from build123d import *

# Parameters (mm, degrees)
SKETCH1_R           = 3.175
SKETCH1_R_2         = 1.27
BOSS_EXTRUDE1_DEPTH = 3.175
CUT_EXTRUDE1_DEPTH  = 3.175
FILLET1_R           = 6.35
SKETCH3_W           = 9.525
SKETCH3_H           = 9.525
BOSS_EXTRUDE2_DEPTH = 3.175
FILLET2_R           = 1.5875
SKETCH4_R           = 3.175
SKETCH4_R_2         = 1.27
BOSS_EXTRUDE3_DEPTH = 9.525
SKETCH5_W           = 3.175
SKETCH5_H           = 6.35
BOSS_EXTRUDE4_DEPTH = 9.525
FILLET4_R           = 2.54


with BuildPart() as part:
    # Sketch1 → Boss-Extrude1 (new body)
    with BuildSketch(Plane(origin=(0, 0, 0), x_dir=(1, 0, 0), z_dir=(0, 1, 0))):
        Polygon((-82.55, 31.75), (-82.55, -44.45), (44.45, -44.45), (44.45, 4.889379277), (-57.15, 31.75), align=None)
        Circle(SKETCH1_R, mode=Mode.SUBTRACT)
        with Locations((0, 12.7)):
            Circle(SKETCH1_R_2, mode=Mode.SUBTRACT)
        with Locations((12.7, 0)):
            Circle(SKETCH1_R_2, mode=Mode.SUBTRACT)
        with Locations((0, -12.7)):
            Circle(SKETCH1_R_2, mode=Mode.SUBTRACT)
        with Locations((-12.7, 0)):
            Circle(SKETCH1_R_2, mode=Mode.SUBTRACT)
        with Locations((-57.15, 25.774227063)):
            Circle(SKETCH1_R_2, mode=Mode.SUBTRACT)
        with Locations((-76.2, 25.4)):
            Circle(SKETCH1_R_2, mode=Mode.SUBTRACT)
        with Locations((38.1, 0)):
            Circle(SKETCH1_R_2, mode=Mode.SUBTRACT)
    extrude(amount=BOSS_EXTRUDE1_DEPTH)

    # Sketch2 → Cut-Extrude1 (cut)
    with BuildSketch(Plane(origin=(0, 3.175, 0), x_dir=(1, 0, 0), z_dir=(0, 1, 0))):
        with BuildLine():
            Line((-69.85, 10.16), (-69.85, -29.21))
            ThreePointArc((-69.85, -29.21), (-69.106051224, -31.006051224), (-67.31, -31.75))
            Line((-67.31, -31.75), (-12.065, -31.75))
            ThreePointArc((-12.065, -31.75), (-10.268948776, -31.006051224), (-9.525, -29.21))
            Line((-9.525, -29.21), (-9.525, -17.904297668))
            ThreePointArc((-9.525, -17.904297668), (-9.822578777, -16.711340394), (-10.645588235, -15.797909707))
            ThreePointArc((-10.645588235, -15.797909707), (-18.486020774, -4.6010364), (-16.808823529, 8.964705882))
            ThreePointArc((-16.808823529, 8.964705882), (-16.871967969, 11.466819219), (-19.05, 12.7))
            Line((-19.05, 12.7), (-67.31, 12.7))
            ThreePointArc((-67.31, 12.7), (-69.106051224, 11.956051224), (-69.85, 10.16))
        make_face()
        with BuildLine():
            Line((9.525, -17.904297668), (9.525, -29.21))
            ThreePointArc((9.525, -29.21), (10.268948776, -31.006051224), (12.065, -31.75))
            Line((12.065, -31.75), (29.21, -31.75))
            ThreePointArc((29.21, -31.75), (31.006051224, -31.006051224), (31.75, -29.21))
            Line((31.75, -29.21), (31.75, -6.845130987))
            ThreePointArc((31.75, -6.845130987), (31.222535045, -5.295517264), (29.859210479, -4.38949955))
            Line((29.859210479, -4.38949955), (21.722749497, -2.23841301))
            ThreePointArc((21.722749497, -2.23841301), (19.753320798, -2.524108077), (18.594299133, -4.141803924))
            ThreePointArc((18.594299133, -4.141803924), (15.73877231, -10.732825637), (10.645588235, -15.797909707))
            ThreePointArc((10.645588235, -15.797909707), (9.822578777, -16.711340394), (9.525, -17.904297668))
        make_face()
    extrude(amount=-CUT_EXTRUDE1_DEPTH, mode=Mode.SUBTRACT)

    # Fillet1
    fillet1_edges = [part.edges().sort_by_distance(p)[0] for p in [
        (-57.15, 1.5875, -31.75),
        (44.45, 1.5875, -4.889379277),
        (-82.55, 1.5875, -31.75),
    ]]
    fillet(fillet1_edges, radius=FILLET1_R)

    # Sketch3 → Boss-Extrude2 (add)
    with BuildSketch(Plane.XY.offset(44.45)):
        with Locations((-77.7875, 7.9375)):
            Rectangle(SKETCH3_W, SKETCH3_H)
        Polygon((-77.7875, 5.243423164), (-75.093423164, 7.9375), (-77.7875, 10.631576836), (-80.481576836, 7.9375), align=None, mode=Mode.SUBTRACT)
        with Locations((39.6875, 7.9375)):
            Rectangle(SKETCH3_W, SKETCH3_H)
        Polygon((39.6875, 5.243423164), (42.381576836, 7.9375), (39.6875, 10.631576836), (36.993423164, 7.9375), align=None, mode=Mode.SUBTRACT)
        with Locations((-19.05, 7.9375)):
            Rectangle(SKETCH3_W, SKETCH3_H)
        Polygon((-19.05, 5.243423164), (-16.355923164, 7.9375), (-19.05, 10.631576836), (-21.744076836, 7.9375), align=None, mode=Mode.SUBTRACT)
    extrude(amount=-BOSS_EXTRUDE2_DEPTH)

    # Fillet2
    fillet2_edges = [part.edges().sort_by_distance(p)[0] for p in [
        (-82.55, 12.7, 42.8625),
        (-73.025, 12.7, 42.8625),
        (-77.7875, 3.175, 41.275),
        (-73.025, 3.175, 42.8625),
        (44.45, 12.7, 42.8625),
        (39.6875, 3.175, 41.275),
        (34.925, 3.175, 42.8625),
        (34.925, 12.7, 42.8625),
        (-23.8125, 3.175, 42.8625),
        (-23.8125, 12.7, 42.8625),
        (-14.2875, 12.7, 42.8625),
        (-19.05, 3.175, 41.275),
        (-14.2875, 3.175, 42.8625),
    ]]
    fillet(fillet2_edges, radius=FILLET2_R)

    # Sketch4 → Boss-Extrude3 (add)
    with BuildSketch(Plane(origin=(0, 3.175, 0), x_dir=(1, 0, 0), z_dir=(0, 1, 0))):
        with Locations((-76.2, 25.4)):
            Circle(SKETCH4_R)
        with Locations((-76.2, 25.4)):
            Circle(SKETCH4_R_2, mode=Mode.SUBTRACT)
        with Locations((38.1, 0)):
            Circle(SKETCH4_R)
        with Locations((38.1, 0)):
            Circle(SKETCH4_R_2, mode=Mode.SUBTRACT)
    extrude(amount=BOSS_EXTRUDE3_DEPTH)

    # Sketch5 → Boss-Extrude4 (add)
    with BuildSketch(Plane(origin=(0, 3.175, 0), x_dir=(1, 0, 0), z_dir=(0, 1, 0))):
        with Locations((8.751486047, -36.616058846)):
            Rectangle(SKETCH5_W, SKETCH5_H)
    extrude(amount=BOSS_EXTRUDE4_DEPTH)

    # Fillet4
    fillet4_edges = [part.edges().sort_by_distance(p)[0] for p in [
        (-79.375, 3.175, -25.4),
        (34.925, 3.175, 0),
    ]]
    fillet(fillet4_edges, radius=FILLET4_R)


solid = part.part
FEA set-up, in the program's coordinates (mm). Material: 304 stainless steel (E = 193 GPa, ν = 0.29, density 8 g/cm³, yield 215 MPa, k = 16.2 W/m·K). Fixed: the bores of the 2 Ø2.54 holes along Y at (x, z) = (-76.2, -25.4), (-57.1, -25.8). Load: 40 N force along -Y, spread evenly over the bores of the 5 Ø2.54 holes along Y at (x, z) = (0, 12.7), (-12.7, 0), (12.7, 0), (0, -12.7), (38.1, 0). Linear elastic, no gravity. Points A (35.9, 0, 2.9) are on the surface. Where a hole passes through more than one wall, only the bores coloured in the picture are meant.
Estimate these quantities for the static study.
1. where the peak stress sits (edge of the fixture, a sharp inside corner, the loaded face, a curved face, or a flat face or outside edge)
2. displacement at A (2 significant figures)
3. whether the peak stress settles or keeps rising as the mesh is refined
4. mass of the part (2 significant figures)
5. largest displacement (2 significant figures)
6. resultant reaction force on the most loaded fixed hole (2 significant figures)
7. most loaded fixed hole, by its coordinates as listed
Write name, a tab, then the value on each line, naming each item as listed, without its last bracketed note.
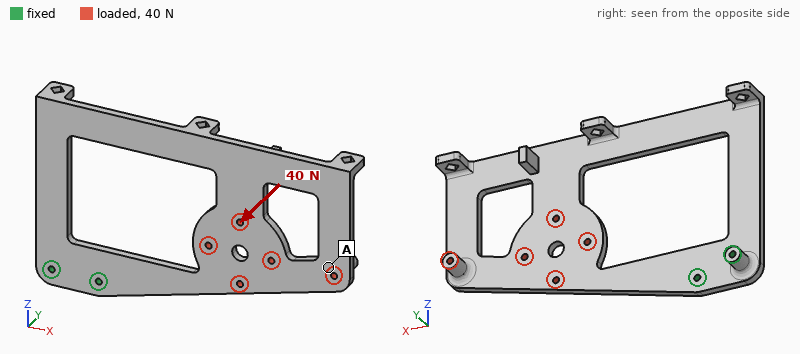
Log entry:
where the peak stress sits	edge of the fixture
displacement at A	0.88 mm
whether the peak stress settles or keeps rising as the mesh is refined	keeps rising
mass of the part	140 g
largest displacement	1.1 mm
resultant reaction force on the most loaded fixed hole	120 N
most loaded fixed hole, by its coordinates as listed	(-57.1, -25.8)
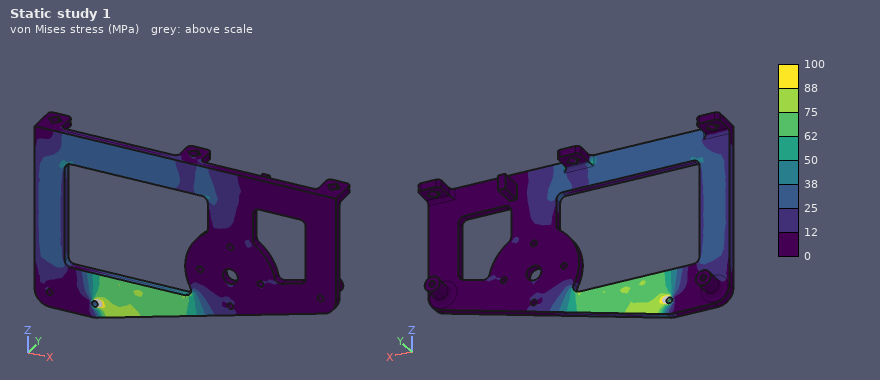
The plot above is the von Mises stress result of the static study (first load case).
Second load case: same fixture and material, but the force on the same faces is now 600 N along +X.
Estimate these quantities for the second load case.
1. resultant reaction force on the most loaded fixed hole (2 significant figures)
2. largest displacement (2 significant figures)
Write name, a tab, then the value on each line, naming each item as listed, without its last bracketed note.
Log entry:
resultant reaction force on the most loaded fixed hole	790 N
largest displacement	0.71 mm
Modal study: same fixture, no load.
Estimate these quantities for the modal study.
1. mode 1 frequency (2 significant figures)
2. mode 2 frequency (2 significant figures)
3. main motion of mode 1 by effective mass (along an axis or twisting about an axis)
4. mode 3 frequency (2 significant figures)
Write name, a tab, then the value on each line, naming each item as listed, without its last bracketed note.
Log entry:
mode 1 frequency	130 Hz
mode 2 frequency	350 Hz
main motion of mode 1 by effective mass	along Y
mode 3 frequency	780 Hz
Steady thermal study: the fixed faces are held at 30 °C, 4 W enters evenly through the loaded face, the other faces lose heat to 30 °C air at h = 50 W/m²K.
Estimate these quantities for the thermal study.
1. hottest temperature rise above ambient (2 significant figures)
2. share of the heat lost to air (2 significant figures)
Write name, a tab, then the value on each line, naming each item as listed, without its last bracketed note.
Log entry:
hottest temperature rise above ambient	39 K
share of the heat lost to air	99 %
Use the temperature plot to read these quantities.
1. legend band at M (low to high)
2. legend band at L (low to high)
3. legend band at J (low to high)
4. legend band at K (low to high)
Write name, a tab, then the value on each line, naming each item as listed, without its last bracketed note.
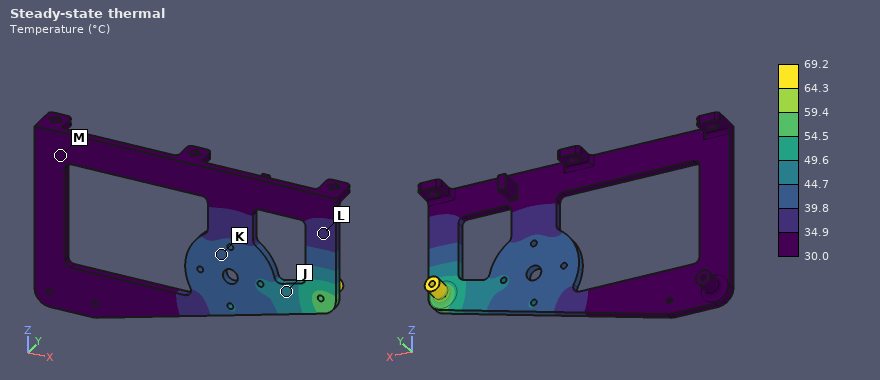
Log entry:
legend band at M	30.0 to 34.9 °C
legend band at L	34.9 to 39.8 °C
legend band at J	44.7 to 49.6 °C
legend band at K	39.8 to 44.7 °C
